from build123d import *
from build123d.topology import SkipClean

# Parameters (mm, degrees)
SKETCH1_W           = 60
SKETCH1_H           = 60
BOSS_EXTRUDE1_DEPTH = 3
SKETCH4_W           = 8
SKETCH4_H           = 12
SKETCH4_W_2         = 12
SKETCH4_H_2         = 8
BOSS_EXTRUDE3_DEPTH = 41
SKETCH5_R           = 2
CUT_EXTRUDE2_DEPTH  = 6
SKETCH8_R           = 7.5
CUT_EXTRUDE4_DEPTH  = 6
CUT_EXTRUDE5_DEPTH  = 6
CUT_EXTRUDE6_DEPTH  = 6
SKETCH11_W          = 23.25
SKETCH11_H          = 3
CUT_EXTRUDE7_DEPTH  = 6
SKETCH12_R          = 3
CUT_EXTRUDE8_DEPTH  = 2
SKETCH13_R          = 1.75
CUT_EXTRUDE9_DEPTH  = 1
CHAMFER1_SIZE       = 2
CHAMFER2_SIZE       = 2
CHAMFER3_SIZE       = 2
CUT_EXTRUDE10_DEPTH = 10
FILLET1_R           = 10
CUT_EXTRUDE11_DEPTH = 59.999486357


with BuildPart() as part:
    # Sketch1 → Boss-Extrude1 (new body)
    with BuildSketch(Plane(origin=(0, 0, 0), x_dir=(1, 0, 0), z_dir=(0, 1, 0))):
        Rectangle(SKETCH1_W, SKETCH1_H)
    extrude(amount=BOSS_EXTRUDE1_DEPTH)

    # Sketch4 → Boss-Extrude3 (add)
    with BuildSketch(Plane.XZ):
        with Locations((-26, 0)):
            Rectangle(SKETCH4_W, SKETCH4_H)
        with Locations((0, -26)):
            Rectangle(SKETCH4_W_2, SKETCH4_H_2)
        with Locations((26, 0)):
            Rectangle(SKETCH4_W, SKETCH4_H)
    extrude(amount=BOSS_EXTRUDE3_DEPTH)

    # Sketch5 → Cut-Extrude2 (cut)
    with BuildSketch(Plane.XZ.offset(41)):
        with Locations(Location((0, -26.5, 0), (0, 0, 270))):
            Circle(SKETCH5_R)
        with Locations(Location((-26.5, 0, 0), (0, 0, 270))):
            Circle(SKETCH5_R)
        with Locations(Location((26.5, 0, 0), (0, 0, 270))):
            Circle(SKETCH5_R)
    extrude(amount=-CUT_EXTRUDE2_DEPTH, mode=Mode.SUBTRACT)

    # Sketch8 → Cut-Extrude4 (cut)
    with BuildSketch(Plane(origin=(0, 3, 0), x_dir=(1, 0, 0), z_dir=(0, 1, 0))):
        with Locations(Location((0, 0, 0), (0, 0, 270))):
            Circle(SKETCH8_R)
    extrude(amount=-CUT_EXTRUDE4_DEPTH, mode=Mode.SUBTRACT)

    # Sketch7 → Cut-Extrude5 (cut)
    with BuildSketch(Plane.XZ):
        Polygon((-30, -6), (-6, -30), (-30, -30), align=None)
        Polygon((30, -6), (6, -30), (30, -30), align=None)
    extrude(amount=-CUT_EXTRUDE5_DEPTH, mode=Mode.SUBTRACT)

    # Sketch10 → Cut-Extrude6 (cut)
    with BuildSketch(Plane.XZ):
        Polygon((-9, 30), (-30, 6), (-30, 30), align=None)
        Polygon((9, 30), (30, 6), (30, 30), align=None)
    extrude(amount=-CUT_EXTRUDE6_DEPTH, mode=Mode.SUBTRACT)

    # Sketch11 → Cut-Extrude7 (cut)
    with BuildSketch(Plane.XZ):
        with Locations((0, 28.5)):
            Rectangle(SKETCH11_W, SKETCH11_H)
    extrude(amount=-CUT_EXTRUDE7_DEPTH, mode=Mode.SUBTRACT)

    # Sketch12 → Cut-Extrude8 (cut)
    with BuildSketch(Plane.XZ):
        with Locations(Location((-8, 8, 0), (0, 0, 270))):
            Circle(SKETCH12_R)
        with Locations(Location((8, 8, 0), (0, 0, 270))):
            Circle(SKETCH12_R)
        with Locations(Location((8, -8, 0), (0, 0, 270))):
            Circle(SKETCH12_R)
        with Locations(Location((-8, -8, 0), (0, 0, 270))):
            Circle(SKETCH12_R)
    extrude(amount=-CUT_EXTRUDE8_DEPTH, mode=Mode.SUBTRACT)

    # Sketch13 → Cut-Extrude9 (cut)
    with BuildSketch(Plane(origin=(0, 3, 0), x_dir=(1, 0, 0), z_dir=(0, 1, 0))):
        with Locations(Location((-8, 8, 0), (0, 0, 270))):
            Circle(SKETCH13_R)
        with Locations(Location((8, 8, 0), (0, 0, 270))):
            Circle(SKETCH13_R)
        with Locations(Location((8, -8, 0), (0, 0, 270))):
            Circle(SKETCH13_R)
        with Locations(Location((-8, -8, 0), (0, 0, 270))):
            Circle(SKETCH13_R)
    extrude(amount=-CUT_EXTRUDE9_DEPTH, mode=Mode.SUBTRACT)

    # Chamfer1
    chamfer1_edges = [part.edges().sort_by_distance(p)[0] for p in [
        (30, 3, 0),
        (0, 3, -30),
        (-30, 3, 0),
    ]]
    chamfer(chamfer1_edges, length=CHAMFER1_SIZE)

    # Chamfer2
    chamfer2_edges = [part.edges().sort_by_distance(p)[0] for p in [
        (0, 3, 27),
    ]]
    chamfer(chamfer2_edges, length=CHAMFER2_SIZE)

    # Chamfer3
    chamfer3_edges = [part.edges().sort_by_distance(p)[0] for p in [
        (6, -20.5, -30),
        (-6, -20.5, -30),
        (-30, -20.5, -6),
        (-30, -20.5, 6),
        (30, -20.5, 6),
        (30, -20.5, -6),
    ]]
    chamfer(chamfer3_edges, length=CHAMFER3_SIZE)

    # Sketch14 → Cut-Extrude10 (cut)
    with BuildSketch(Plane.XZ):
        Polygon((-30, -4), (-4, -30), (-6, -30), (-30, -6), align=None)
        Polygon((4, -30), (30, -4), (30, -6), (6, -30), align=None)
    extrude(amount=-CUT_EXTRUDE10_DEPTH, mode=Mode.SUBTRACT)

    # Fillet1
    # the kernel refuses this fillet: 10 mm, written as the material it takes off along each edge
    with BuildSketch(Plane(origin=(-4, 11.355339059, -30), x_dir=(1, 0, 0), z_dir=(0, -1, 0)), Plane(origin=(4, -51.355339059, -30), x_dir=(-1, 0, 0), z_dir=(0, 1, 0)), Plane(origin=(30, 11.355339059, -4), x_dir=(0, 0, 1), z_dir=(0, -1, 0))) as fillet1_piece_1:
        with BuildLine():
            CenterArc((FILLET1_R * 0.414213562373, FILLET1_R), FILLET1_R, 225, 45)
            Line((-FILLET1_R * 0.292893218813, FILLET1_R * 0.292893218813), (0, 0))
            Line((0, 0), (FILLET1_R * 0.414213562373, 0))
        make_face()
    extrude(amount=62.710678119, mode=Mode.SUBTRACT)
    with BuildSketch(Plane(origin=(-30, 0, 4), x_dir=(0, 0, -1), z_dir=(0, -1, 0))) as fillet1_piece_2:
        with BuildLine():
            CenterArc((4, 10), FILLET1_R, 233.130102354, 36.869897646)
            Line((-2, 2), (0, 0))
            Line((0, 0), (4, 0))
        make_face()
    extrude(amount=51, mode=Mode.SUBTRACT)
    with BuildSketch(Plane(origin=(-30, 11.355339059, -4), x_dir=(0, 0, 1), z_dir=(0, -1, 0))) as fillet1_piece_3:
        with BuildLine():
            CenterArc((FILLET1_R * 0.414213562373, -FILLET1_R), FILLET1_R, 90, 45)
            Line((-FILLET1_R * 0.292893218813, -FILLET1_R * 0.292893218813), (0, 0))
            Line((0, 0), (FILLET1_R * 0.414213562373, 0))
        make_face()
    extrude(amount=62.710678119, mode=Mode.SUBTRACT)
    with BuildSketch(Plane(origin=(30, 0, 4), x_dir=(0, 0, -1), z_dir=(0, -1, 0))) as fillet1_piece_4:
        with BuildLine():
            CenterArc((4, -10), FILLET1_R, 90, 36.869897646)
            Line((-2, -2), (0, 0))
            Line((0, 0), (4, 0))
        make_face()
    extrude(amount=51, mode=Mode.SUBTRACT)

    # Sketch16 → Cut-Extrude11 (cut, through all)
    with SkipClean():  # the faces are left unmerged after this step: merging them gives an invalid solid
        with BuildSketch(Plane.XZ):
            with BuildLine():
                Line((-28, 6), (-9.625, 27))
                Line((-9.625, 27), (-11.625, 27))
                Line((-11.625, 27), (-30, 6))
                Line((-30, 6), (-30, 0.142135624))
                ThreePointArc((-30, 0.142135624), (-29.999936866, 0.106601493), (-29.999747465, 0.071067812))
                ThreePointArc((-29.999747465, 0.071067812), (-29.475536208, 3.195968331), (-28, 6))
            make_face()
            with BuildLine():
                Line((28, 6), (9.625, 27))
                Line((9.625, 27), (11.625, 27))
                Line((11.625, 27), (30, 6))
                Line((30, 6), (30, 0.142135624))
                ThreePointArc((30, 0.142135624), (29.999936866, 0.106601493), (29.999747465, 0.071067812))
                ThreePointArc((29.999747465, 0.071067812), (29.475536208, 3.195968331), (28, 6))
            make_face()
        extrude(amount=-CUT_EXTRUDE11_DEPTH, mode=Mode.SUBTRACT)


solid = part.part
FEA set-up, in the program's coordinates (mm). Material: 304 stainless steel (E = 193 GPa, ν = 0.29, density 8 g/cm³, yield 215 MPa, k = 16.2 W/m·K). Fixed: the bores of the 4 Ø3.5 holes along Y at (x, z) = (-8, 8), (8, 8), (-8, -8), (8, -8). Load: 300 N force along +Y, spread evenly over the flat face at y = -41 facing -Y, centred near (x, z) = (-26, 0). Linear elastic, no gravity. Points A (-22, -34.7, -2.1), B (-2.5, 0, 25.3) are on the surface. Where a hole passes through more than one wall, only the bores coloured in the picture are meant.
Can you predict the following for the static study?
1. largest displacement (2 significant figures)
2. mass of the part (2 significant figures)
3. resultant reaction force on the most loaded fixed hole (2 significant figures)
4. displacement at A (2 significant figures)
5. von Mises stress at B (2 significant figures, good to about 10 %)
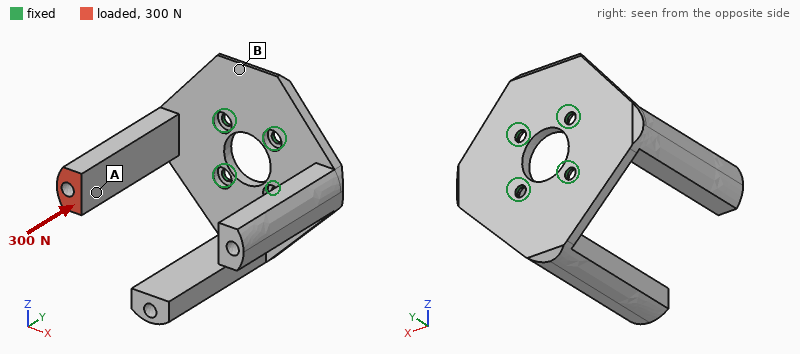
0.22 mm
130 g
390 N
0.18 mm
21 MPa
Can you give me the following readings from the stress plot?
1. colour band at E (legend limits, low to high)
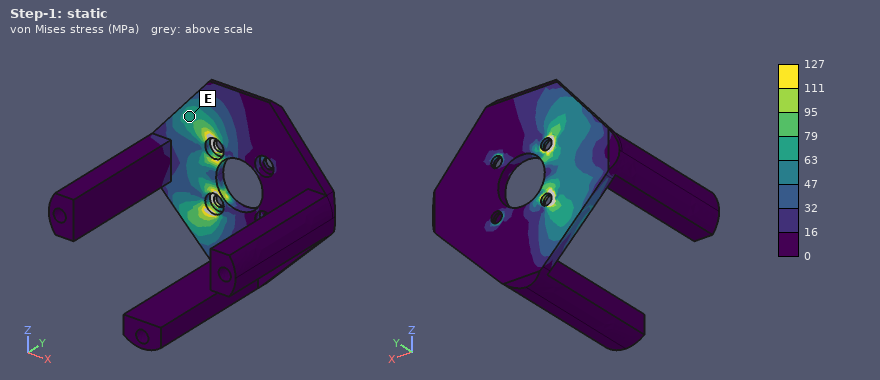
63 to 79 MPa
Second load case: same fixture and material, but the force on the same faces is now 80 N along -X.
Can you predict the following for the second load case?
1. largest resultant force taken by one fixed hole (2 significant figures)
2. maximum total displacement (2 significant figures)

230 N
0.26 mm
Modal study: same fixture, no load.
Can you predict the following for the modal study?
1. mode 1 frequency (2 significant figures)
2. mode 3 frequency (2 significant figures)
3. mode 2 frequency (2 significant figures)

830 Hz
900 Hz
870 Hz
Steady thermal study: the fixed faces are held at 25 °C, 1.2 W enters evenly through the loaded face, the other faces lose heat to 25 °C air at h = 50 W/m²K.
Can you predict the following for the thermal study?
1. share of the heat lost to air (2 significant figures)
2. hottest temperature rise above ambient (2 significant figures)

86 %
22 K
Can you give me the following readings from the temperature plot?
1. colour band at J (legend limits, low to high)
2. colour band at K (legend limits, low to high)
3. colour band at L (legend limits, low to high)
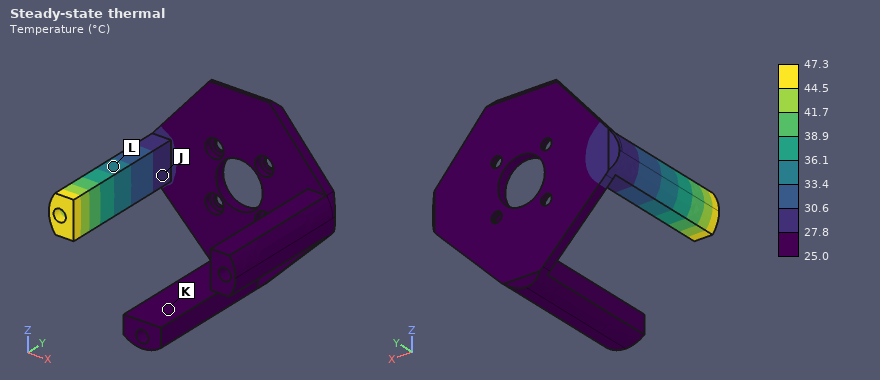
27.8 to 30.6 °C
25.0 to 27.8 °C
33.4 to 36.1 °C
